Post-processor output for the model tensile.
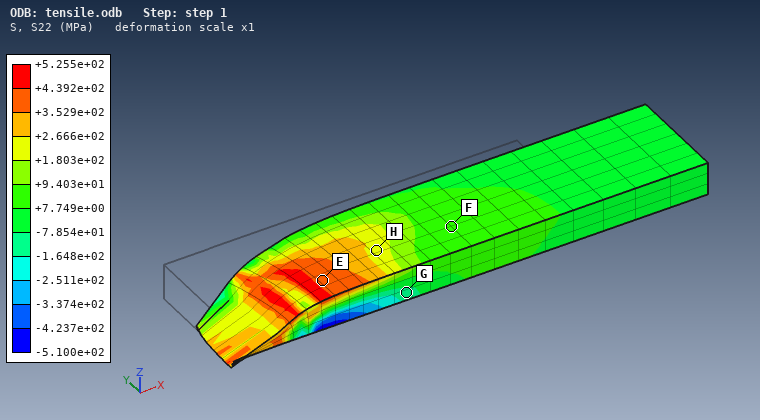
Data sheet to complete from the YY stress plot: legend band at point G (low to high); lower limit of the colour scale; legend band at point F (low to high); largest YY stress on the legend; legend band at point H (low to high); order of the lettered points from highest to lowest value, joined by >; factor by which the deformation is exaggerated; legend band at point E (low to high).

-1.648e+02 to -7.854e+01 MPa
-5.100e+02 MPa
+7.749e+00 to +9.403e+01 MPa
+5.255e+02 MPa
+1.803e+02 to +2.666e+02 MPa
E > H > F > G
1
+3.529e+02 to +4.392e+02 MPa
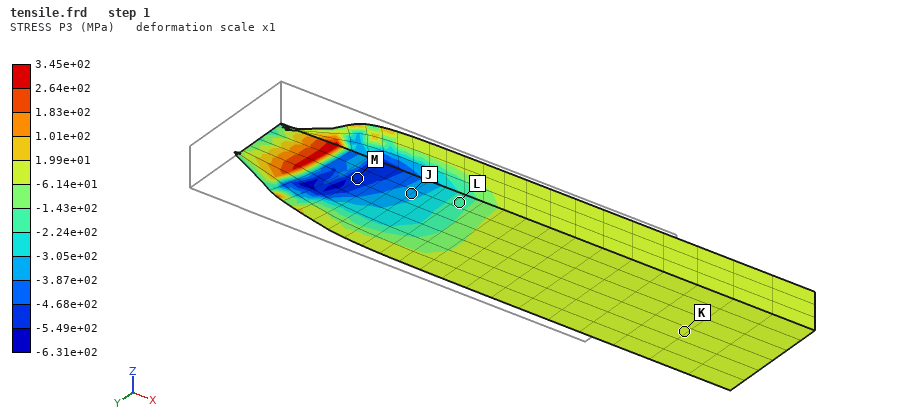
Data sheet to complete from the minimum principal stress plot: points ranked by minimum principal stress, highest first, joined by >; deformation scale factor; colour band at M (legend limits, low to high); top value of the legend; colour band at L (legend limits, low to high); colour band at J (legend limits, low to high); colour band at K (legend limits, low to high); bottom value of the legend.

K > L > J > M
1
-5.49e+02 to -4.68e+02 MPa
3.45e+02 MPa
-2.24e+02 to -1.43e+02 MPa
-3.87e+02 to -3.05e+02 MPa
-6.14e+01 to 1.99e+01 MPa
-6.31e+02 MPa
